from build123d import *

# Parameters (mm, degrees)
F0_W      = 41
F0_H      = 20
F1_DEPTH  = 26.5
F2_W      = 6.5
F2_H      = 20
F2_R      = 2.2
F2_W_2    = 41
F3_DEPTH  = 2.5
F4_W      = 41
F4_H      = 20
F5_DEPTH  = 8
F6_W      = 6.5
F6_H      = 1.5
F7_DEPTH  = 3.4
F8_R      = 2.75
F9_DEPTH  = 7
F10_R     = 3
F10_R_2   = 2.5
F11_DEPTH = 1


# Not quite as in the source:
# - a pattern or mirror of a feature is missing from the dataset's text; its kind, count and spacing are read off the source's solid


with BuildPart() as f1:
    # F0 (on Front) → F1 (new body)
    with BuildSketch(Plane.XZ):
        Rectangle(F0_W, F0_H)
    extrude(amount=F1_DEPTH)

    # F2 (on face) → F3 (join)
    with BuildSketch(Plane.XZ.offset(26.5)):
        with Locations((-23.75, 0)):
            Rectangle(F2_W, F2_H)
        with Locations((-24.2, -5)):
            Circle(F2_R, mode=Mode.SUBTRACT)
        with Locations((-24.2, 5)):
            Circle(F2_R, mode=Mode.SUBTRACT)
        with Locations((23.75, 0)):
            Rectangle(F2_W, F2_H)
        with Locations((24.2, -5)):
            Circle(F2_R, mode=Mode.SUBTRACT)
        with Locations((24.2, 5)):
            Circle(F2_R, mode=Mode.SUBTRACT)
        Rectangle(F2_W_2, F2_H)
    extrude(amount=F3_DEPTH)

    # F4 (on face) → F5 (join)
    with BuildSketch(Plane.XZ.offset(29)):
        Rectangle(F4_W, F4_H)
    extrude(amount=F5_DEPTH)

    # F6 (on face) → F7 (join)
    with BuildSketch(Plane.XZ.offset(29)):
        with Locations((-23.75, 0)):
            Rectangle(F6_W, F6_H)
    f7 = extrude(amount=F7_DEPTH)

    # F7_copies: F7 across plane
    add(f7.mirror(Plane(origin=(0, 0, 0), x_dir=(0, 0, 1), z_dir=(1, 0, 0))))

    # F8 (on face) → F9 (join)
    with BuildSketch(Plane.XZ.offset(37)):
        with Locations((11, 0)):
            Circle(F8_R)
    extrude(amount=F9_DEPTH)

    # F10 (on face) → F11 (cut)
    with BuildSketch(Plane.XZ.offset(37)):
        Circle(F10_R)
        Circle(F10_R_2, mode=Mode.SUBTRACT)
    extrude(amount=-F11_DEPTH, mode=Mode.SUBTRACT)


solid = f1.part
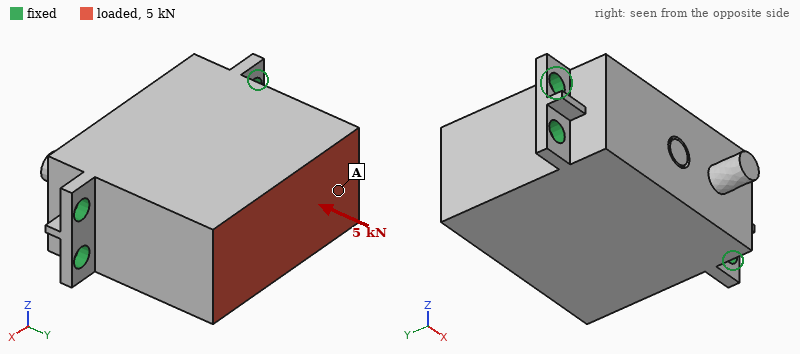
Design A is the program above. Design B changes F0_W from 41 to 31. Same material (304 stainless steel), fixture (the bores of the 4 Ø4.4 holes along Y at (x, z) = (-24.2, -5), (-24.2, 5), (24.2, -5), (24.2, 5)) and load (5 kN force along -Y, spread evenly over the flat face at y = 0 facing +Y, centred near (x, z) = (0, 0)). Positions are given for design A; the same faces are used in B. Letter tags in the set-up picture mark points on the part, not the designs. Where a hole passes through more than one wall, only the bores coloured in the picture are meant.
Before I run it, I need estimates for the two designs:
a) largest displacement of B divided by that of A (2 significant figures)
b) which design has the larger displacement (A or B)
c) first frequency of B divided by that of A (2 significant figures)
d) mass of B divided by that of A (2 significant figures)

1.8
B
0.88
0.83
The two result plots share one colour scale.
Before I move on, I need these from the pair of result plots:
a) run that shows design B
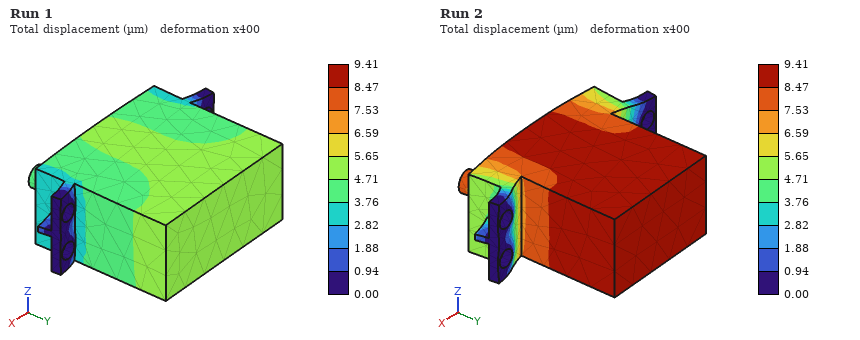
Run 2
